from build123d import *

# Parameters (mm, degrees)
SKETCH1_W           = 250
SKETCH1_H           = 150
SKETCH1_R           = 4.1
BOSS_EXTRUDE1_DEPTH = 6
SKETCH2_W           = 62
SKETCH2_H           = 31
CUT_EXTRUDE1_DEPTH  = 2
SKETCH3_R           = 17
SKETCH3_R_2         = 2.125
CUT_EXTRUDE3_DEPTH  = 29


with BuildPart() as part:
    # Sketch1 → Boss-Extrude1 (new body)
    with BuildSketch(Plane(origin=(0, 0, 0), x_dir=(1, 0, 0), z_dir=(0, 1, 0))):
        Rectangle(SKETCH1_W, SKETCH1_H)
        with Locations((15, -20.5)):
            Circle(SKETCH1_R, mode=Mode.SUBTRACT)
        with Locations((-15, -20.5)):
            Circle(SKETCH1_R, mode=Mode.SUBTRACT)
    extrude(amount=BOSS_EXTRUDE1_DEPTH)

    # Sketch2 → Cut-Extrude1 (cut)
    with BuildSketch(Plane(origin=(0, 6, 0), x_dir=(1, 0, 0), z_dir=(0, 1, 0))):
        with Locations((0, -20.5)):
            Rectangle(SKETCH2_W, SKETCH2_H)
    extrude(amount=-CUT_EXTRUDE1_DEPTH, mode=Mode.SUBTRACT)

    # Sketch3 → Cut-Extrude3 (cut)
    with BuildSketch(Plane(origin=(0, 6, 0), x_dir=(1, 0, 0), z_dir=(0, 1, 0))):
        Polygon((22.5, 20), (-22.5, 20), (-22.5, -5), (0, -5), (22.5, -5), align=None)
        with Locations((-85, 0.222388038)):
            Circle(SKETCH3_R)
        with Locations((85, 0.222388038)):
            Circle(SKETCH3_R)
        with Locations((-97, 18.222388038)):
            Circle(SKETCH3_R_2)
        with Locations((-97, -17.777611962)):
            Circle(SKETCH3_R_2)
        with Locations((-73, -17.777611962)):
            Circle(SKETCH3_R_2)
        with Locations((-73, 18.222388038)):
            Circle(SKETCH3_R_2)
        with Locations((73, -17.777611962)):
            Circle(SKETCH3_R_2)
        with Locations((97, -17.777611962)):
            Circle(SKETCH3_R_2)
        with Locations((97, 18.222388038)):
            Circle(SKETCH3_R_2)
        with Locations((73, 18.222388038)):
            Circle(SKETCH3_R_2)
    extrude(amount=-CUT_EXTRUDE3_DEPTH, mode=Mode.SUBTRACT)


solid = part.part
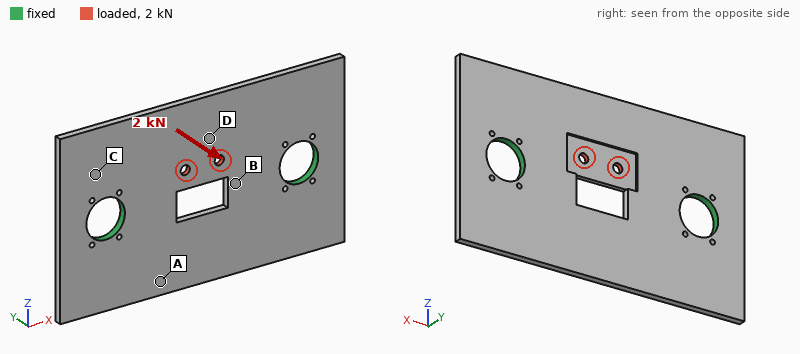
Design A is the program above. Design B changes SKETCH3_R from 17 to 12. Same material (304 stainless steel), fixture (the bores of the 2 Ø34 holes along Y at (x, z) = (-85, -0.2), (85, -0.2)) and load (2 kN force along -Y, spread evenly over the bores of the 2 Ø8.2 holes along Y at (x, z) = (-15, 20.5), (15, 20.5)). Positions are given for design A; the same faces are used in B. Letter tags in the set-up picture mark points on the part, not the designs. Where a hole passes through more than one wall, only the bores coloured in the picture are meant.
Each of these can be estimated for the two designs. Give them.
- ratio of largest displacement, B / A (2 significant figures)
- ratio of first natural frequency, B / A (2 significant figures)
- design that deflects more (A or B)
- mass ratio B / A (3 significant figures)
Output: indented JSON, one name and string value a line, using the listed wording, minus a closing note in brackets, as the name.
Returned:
{
  "ratio of largest displacement, B / A": "1.2",
  "ratio of first natural frequency, B / A": "0.86",
  "design that deflects more": "B",
  "mass ratio B / A": "1.03"
}
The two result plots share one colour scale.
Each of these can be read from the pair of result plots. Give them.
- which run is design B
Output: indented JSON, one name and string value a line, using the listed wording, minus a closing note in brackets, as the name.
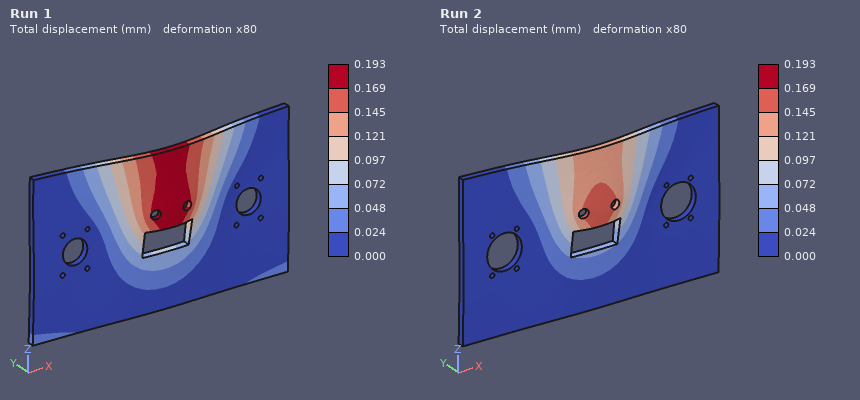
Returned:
{
  "which run is design B": "Run 1"
}
